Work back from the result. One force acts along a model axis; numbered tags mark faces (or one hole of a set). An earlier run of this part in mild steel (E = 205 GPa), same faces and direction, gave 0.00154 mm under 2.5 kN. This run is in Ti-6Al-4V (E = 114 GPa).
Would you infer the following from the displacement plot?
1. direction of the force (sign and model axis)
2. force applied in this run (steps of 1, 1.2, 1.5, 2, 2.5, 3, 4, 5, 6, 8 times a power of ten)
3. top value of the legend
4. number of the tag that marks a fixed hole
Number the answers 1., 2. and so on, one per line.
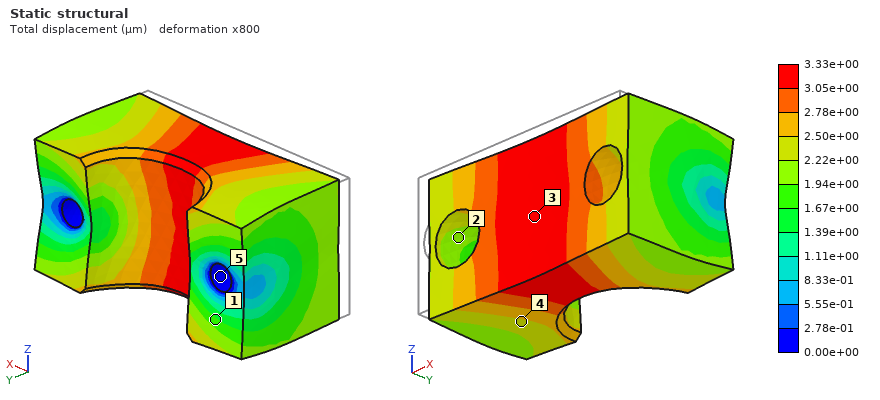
1. +Y
2. 3 kN
3. 3.33e+00 µm
4. 5
